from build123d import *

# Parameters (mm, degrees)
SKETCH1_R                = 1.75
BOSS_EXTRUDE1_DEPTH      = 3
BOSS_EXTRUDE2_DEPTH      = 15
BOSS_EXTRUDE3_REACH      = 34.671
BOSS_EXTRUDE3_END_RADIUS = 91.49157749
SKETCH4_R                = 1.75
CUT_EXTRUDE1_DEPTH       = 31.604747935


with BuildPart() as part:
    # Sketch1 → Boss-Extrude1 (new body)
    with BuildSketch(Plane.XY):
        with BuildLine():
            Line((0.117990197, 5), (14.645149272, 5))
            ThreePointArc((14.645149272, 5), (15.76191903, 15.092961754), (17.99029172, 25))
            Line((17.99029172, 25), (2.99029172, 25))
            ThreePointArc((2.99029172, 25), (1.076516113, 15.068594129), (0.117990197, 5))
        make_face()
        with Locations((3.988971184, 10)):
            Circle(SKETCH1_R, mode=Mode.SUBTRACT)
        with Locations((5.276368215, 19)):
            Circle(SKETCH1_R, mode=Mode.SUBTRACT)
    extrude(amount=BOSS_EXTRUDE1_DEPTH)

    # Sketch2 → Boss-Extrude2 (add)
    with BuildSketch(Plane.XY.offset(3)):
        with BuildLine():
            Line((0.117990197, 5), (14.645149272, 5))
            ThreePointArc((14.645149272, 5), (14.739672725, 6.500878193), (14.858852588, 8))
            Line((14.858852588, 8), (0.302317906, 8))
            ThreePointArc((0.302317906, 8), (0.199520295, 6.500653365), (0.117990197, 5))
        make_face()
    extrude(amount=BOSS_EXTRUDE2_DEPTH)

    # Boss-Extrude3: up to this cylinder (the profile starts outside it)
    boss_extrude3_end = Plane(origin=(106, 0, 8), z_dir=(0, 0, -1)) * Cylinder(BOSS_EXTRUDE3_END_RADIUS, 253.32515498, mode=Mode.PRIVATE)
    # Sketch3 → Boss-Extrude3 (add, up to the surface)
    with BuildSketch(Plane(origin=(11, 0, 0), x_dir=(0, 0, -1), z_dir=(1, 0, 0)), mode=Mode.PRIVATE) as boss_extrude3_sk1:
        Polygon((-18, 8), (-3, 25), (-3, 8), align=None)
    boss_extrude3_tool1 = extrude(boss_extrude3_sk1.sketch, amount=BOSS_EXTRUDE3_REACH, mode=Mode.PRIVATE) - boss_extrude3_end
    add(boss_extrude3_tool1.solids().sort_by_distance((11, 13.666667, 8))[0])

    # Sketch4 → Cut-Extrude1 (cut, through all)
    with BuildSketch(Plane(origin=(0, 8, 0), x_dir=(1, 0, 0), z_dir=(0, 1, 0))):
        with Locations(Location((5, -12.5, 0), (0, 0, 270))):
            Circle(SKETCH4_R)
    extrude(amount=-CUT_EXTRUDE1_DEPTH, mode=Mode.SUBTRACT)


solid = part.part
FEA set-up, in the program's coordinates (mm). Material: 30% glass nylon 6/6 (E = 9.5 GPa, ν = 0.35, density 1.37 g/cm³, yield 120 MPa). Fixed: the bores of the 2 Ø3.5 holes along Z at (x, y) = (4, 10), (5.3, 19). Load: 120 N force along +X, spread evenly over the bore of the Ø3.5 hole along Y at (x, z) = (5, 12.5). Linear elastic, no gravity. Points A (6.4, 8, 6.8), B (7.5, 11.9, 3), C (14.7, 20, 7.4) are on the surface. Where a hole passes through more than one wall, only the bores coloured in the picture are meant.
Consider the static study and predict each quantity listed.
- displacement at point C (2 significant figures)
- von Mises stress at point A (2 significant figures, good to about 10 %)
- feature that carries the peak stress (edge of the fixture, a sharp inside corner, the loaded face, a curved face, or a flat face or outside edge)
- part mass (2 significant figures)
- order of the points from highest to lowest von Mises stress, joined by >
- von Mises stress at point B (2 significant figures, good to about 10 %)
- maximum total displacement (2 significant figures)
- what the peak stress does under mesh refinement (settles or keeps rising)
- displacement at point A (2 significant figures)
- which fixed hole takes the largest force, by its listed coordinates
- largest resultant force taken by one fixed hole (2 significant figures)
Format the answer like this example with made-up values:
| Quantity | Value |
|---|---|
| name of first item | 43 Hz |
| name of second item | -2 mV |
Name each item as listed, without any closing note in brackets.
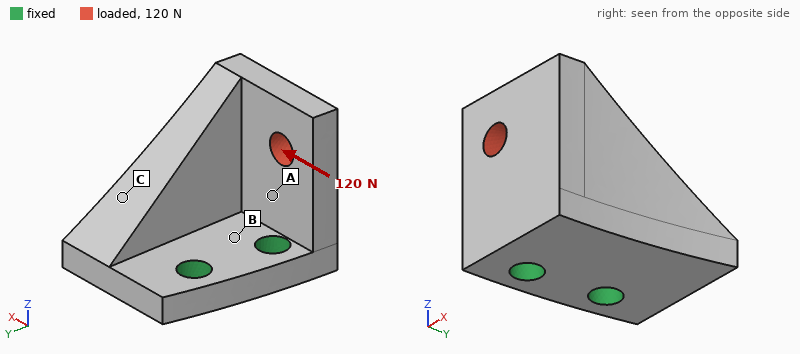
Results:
| Quantity | Value |
|---|---|
| displacement at point C | 0.050 mm |
| von Mises stress at point A | 9.1 MPa |
| feature that carries the peak stress | edge of the fixture |
| part mass | 2.8 g |
| order of the points from highest to lowest von Mises stress, joined by > | B > A > C |
| von Mises stress at point B | 19 MPa |
| maximum total displacement | 0.16 mm |
| what the peak stress does under mesh refinement | keeps rising |
| displacement at point A | 0.044 mm |
| which fixed hole takes the largest force, by its listed coordinates | (4, 10) |
| largest resultant force taken by one fixed hole | 130 N |
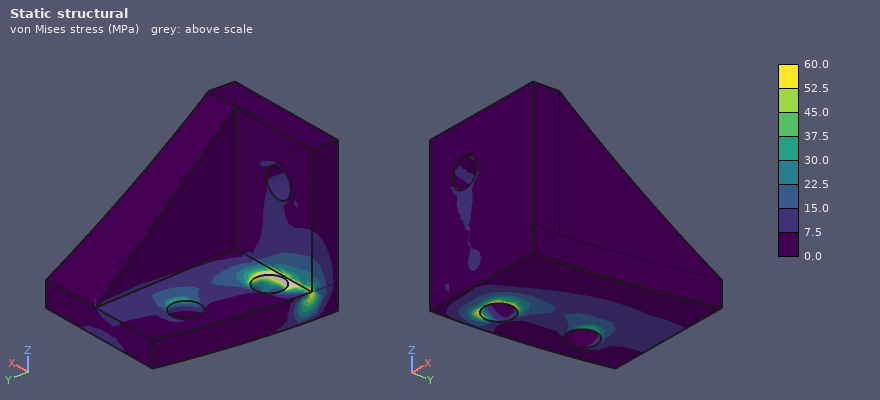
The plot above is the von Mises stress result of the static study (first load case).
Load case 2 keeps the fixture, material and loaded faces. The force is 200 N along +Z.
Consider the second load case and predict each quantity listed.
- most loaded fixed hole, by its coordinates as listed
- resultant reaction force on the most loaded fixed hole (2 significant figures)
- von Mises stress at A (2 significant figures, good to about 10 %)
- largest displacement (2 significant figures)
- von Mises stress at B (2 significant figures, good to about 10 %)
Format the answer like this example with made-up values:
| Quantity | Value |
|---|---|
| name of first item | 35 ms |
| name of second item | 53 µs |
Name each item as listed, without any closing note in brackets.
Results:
| Quantity | Value |
|---|---|
| most loaded fixed hole, by its coordinates as listed | (4, 10) |
| resultant reaction force on the most loaded fixed hole | 210 N |
| von Mises stress at A | 8.9 MPa |
| largest displacement | 43 µm |
| von Mises stress at B | 5.8 MPa |
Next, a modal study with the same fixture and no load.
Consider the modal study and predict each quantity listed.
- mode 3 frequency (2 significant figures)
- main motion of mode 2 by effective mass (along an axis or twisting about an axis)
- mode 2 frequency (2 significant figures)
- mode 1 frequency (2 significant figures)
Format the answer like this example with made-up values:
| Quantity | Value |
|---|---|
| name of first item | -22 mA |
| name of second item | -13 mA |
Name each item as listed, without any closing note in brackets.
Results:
| Quantity | Value |
|---|---|
| mode 3 frequency | 12 kHz |
| main motion of mode 2 by effective mass | along Y |
| mode 2 frequency | 6500 Hz |
| mode 1 frequency | 4600 Hz |
